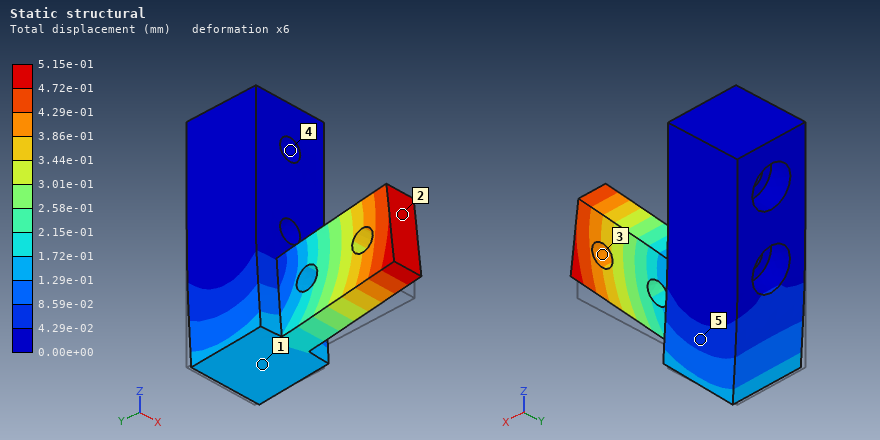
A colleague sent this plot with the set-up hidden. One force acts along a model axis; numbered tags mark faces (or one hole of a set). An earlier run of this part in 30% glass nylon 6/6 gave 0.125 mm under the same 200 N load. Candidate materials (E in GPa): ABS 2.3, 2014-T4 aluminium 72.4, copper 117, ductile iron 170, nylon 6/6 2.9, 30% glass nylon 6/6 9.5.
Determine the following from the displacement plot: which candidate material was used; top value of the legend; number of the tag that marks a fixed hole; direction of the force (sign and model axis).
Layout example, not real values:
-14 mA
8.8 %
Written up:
ABS
5.15e-01 mm
4
+Z
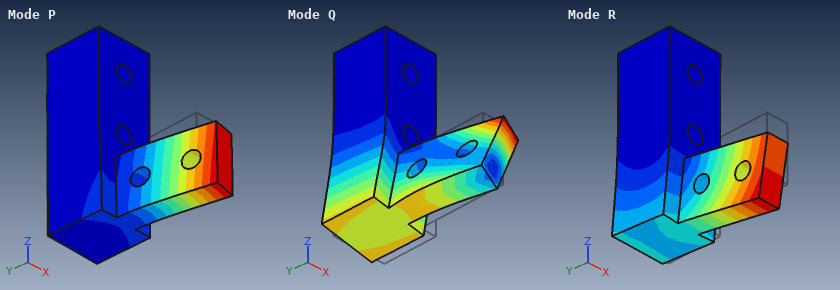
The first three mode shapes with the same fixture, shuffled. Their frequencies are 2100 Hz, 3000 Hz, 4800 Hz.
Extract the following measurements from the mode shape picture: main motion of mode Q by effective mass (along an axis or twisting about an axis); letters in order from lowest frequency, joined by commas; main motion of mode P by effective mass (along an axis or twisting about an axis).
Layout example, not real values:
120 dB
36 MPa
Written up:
along X
P, R, Q
along X
